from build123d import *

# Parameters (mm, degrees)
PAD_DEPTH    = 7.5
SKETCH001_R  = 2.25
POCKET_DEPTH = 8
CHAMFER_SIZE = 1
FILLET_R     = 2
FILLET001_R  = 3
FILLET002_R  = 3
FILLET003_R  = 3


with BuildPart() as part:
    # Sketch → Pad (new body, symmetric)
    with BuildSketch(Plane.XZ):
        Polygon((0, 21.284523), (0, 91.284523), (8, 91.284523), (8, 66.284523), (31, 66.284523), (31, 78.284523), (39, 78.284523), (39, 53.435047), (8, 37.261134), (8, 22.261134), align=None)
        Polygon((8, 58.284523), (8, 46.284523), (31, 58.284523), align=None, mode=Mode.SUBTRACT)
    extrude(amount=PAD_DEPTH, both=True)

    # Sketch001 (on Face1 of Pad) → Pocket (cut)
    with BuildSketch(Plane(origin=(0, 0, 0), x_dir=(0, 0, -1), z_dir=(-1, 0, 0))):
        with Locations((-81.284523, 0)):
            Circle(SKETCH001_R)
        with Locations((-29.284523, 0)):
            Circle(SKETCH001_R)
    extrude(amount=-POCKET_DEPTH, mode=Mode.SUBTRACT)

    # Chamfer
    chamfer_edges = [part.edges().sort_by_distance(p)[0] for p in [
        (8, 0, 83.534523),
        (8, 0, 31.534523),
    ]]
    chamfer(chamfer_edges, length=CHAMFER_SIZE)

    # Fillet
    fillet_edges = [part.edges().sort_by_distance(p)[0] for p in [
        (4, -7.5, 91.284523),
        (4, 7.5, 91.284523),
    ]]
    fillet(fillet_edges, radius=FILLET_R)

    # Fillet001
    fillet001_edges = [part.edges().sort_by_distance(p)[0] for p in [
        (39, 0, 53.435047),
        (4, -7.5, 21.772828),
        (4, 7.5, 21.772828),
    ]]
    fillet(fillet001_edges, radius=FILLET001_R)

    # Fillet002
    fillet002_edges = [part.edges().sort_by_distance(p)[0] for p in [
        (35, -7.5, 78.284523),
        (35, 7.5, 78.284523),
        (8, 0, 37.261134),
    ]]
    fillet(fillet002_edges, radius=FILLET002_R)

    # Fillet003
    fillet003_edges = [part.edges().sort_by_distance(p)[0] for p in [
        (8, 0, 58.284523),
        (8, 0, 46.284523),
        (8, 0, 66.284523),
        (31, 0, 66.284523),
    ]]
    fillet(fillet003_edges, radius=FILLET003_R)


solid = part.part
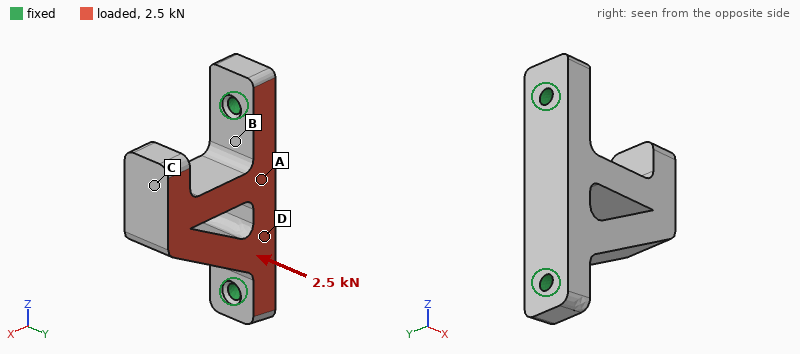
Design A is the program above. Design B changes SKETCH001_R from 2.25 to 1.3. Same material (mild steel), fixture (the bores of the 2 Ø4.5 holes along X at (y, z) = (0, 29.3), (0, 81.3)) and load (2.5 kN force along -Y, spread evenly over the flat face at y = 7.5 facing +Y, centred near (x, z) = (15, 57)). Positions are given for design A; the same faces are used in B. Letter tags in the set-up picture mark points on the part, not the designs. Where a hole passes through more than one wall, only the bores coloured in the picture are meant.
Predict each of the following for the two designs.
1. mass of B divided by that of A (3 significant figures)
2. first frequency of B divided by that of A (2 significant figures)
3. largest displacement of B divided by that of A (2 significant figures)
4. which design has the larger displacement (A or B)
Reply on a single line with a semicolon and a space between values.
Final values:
1.01; 0.91; 1.2; B
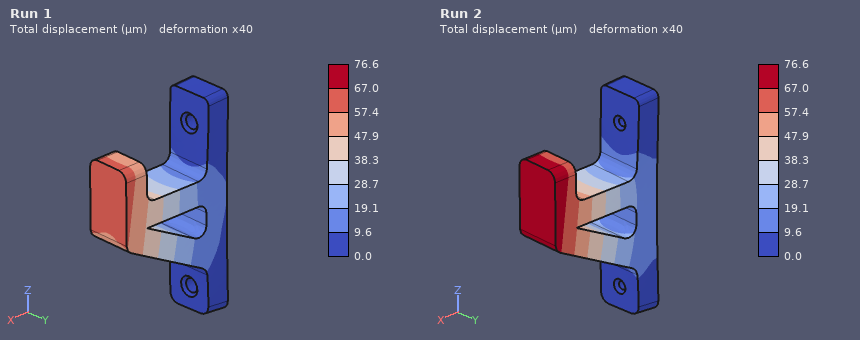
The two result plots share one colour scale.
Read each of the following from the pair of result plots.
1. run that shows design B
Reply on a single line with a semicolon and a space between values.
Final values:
Run 2
